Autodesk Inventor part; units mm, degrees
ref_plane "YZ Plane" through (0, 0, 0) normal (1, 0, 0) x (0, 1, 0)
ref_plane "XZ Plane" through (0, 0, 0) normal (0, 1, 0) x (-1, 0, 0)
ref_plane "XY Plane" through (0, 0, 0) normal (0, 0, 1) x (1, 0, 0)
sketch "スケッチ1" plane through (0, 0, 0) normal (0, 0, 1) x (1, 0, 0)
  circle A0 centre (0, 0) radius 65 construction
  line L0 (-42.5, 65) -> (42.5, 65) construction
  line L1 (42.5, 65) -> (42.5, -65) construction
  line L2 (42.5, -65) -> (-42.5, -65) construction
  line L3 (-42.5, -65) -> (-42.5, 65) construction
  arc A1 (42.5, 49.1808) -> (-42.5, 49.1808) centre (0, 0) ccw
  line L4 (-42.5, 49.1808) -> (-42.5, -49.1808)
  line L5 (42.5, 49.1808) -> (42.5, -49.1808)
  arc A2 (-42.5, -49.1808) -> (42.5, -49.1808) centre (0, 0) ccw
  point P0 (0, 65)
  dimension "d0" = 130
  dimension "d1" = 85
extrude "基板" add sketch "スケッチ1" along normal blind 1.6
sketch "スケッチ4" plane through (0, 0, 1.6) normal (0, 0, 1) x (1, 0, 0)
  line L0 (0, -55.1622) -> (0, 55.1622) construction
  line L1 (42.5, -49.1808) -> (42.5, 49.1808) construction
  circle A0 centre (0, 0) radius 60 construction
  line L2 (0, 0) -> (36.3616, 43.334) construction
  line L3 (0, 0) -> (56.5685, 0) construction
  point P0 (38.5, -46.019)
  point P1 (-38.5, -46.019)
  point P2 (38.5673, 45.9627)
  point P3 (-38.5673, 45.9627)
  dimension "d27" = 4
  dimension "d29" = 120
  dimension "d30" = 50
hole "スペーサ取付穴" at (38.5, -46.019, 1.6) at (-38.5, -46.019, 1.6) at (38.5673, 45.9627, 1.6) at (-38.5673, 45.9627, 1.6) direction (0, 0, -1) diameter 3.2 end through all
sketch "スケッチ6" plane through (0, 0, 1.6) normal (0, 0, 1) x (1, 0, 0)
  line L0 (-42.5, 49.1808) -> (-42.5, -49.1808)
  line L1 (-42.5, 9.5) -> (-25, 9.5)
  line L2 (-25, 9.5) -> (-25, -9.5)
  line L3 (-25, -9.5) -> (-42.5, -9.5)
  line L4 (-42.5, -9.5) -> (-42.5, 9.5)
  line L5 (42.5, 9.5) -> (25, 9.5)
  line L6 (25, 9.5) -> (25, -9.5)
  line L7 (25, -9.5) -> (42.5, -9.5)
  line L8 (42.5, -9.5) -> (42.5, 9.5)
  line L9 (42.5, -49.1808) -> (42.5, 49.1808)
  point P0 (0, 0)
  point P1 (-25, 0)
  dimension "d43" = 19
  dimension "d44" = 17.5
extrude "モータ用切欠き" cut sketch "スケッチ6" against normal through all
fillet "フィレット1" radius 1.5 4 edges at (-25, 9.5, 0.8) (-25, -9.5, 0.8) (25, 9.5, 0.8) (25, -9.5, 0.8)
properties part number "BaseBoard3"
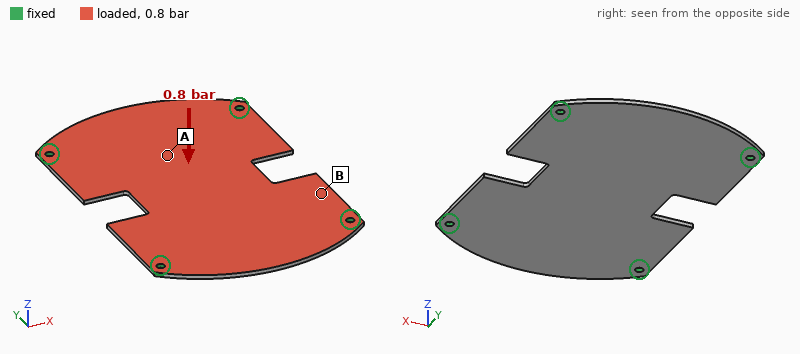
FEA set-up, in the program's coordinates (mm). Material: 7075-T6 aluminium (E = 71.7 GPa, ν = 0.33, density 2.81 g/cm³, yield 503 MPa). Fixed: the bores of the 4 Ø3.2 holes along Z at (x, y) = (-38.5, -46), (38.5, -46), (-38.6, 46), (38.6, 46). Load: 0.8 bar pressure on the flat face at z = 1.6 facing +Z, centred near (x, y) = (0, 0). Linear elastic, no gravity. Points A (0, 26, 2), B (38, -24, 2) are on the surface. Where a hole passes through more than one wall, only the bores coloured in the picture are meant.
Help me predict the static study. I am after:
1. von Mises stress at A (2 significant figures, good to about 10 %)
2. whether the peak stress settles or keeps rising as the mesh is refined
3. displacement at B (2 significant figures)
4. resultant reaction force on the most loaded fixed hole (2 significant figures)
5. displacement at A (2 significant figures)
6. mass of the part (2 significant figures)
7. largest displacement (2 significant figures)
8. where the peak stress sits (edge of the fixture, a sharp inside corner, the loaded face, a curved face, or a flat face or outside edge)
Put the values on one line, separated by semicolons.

59 MPa; keeps rising; 0.51 mm; 190 N; 0.95 mm; 43 g; 1.3 mm; edge of the fixture
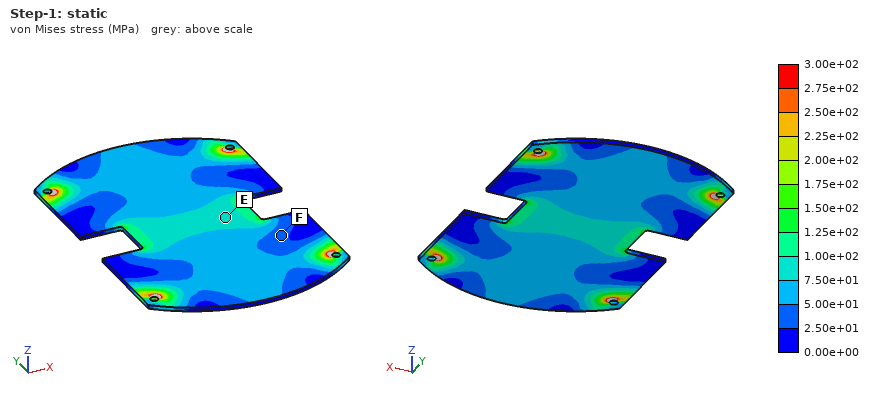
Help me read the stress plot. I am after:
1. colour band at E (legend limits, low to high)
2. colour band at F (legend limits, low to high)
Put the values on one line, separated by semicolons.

7.50e+01 to 1.00e+02 MPa; 2.50e+01 to 5.00e+01 MPa
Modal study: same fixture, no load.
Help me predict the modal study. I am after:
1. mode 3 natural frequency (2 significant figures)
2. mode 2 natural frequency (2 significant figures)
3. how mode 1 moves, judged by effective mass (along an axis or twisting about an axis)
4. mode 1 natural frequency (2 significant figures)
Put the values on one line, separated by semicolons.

1300 Hz; 1200 Hz; along Z; 690 Hz
